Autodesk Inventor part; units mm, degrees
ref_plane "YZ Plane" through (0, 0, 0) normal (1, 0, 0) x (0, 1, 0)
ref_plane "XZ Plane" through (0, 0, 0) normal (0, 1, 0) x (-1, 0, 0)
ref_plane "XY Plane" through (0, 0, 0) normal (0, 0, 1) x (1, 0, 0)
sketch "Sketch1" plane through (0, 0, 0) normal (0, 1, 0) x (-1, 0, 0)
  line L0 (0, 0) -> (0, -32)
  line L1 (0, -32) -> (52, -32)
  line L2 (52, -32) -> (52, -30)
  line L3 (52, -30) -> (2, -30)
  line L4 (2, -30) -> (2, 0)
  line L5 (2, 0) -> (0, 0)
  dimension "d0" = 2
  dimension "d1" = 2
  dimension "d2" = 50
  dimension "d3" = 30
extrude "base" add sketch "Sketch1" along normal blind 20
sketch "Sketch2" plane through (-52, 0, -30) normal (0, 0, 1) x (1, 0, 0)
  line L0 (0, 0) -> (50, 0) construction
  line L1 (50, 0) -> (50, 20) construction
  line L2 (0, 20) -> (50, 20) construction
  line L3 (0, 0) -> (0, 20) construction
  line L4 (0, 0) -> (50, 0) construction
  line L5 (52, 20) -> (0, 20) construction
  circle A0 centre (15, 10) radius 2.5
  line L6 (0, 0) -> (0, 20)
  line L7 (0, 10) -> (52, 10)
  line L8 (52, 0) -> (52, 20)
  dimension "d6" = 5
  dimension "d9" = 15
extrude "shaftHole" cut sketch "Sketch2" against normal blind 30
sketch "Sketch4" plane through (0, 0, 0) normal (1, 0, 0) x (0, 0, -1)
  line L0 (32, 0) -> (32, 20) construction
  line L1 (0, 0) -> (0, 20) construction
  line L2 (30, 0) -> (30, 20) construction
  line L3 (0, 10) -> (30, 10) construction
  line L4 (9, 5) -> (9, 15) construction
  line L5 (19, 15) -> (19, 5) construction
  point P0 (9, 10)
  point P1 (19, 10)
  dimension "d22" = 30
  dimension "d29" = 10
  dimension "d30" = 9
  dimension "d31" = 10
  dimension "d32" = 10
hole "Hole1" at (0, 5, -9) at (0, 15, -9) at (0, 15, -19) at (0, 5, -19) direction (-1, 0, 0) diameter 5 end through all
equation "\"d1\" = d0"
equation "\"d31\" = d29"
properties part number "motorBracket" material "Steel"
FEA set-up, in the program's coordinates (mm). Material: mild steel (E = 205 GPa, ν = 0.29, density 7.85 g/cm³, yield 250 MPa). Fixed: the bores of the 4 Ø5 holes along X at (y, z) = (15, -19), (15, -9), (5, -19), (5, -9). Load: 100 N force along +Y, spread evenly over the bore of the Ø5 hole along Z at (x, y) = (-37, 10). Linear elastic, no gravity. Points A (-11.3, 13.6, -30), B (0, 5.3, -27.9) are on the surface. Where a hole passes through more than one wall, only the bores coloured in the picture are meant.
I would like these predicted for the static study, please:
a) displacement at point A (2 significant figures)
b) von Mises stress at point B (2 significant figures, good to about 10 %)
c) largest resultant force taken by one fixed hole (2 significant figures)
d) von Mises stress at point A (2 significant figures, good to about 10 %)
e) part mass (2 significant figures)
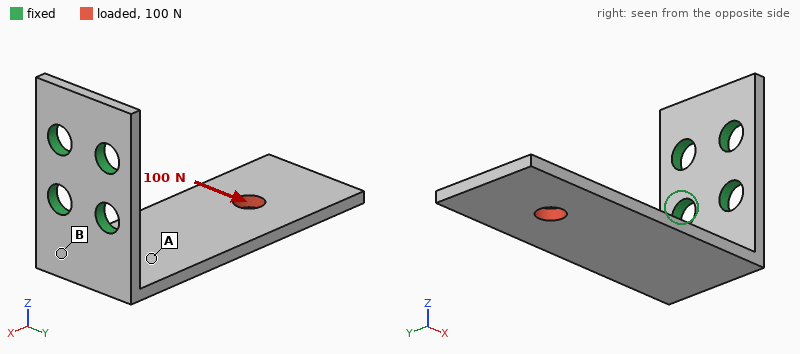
0.045 mm
120 MPa
290 N
22 MPa
24 g
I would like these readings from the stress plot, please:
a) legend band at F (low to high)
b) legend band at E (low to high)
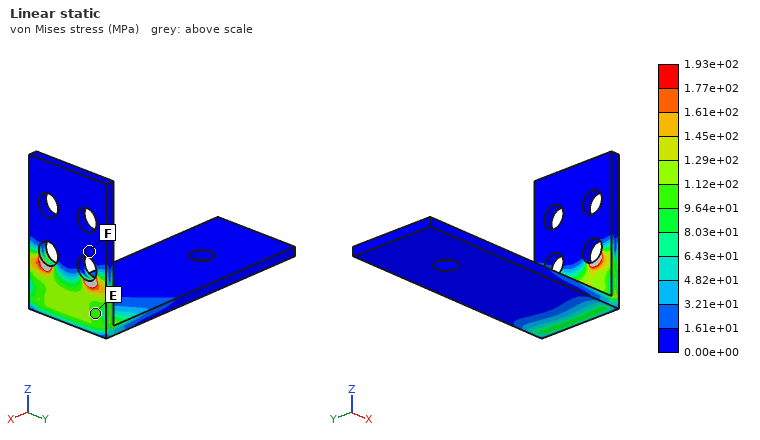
0.00e+00 to 1.61e+01 MPa
9.64e+01 to 1.12e+02 MPa
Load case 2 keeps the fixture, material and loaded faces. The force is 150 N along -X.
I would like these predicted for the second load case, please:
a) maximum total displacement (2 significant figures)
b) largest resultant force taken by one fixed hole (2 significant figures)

0.14 mm
76 N
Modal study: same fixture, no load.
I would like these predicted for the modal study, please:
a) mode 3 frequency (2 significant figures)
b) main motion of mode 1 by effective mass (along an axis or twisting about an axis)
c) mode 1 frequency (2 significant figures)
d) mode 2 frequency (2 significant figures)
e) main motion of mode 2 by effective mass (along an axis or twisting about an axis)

3000 Hz
along Z
500 Hz
1300 Hz
along Y
